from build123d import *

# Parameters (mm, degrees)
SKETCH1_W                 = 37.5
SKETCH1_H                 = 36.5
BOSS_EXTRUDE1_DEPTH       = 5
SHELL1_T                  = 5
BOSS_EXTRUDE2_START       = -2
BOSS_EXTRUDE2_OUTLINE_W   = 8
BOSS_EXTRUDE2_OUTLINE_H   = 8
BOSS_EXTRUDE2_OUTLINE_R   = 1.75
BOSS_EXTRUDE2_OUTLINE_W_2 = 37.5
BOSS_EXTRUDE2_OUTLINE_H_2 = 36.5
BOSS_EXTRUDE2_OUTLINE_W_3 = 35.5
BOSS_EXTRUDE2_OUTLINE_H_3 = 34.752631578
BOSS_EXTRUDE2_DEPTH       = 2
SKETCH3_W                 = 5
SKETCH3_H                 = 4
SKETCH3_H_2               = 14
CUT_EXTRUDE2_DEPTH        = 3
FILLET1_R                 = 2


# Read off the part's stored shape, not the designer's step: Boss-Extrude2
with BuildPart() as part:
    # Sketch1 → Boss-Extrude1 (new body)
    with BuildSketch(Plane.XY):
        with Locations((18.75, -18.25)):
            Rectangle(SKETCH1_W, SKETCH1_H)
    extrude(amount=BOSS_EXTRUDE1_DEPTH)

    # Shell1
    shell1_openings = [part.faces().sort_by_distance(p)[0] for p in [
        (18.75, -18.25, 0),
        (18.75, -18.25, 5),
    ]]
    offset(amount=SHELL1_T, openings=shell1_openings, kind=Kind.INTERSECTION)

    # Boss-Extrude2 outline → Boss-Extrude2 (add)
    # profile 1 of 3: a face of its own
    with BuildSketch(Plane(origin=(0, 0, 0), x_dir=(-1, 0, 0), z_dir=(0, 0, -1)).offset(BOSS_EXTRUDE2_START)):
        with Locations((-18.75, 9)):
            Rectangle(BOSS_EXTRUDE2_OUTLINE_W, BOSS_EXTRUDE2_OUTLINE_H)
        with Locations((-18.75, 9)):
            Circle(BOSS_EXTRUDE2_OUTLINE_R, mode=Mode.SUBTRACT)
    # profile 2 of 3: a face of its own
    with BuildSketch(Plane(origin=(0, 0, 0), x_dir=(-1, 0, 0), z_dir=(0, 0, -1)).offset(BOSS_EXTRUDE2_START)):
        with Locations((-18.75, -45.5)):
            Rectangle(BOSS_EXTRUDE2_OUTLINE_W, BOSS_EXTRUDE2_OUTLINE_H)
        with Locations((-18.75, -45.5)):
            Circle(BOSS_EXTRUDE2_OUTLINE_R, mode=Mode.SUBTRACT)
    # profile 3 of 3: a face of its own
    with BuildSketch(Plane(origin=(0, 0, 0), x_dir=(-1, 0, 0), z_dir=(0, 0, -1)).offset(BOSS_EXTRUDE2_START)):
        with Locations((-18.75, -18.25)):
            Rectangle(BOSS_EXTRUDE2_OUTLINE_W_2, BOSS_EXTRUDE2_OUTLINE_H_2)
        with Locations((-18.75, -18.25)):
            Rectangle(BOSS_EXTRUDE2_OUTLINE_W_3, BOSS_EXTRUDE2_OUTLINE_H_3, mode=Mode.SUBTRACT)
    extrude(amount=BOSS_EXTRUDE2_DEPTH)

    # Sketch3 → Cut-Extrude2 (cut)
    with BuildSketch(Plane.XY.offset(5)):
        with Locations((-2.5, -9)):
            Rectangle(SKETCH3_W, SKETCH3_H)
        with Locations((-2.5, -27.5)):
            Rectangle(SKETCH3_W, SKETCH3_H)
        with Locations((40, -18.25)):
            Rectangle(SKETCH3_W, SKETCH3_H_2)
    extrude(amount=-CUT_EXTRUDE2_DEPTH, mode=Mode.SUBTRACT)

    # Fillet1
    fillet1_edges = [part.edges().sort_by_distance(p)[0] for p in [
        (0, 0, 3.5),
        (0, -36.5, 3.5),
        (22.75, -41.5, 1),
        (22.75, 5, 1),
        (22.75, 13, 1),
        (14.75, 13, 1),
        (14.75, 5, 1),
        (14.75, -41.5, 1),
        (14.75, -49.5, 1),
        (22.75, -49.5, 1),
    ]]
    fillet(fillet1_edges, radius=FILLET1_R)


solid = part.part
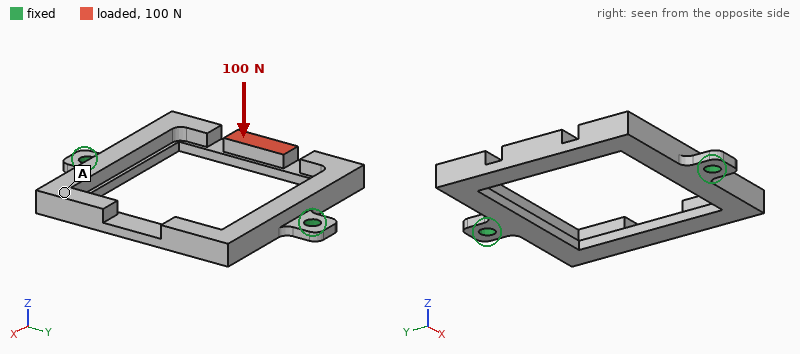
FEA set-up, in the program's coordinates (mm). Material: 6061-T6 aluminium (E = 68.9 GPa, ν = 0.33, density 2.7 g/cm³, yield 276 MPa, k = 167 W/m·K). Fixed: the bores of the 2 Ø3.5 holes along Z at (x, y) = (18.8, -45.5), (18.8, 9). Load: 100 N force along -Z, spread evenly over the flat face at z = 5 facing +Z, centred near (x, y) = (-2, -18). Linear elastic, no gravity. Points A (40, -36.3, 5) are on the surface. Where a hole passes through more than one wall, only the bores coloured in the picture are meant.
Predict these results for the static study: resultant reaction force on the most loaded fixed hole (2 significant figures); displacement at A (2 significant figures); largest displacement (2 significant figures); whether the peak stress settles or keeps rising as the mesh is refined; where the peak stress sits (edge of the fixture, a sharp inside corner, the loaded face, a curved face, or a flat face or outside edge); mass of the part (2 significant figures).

50 N
0.082 mm
0.26 mm
keeps rising
edge of the fixture
12 g
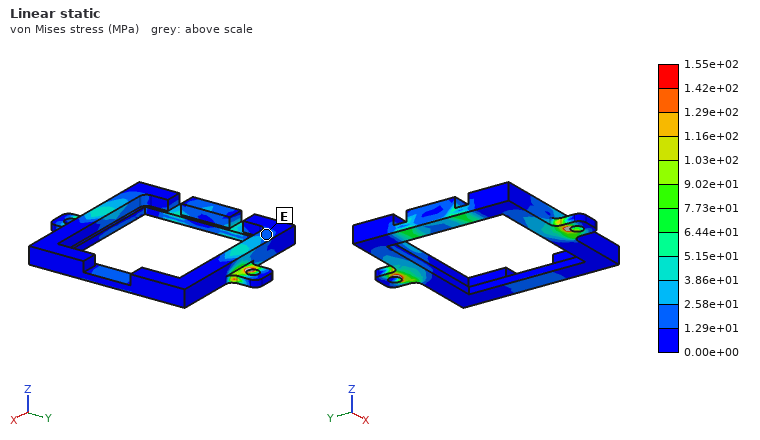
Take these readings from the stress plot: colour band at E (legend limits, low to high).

1.29e+01 to 2.58e+01 MPa
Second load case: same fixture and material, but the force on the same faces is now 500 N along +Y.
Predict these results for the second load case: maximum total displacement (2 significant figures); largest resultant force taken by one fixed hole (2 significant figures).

0.15 mm
290 N
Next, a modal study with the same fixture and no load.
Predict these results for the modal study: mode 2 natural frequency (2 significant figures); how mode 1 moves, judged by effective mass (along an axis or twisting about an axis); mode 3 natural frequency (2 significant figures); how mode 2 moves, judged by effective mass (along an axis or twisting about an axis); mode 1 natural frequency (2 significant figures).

2600 Hz
twisting about Y
3600 Hz
along Z
1700 Hz
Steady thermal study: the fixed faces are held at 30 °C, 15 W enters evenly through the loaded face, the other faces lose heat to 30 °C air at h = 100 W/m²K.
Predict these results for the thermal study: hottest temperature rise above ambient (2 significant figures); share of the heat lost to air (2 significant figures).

64 K
40 %
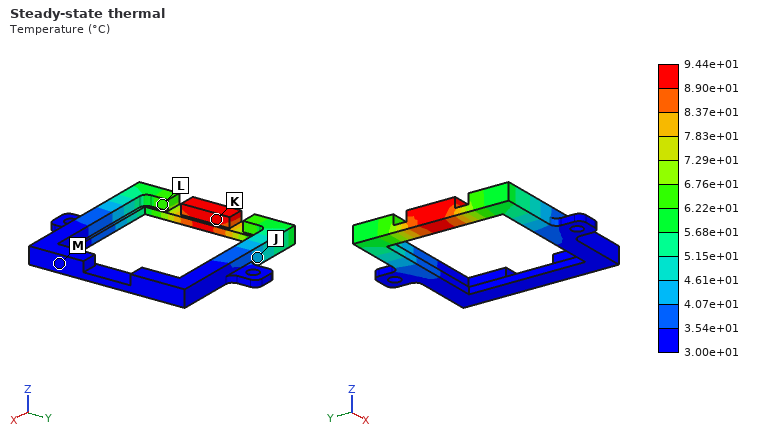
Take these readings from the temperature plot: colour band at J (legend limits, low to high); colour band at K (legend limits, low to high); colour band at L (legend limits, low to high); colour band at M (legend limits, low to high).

4.07e+01 to 4.61e+01 °C
8.90e+01 to 9.44e+01 °C
6.22e+01 to 6.76e+01 °C
3.00e+01 to 3.54e+01 °C
